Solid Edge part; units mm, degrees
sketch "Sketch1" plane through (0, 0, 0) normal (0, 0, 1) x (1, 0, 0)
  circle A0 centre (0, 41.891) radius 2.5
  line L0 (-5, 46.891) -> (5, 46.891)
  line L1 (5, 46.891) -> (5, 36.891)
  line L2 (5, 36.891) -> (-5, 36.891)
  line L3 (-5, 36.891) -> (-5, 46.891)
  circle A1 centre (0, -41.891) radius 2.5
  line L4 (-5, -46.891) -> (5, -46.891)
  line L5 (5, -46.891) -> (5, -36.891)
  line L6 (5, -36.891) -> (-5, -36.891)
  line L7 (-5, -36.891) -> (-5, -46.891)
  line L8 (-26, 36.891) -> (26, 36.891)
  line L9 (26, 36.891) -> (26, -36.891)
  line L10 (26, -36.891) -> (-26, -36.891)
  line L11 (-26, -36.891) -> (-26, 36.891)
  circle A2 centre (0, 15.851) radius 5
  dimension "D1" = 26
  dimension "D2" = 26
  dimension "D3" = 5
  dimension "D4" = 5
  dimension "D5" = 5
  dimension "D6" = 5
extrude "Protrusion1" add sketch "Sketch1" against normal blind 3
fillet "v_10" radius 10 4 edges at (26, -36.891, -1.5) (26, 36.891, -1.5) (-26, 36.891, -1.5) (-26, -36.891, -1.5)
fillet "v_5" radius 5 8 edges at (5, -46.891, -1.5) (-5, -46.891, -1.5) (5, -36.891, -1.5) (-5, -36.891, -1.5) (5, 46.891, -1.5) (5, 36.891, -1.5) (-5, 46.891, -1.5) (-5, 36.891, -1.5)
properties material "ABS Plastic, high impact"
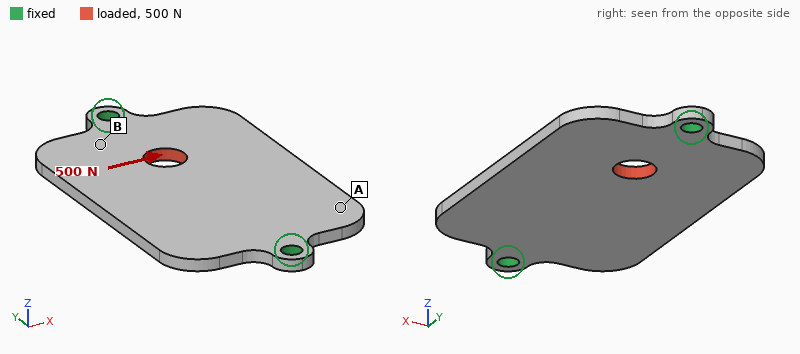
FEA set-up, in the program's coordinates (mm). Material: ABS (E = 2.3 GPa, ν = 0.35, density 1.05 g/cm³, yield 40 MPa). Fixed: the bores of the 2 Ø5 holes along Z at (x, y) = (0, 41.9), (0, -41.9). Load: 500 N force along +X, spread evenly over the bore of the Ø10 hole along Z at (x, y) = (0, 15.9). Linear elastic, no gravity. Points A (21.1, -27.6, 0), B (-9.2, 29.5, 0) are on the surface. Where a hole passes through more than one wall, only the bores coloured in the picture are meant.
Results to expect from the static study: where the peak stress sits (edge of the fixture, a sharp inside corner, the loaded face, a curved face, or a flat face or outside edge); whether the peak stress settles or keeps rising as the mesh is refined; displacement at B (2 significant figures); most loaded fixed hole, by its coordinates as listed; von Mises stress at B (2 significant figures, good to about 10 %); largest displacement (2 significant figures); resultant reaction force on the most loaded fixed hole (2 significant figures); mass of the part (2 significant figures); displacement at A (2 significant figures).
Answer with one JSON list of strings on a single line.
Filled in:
["edge of the fixture", "keeps rising", "0.11 mm", "(0, 41.9)", "6.4 MPa", "0.18 mm", "350 N", "12 g", "0.079 mm"]
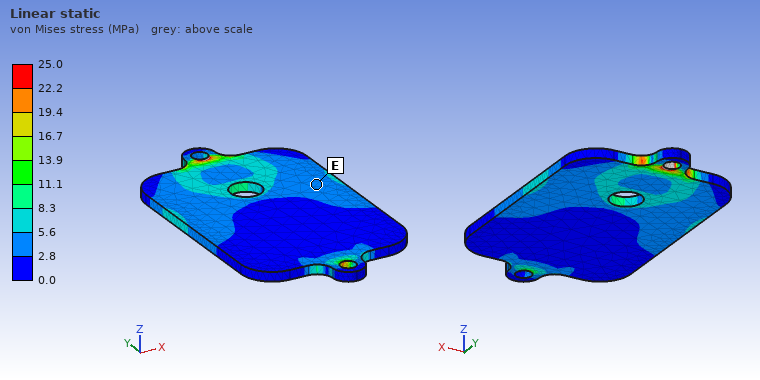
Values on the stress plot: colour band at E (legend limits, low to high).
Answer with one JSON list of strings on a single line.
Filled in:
["2.8 to 5.6 MPa"]
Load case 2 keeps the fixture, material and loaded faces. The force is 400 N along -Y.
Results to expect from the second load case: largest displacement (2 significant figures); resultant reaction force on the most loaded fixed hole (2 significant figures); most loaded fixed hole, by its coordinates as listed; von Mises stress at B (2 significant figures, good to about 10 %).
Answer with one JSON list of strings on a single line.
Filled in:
["62 µm", "240 N", "(0, 41.9)", "2.3 MPa"]
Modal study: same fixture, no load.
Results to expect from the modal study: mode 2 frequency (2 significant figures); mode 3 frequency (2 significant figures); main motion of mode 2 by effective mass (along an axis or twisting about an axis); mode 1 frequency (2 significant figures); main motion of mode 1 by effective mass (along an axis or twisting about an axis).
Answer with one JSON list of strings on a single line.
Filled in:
["470 Hz", "1100 Hz", "along Z", "420 Hz", "twisting about Y"]
